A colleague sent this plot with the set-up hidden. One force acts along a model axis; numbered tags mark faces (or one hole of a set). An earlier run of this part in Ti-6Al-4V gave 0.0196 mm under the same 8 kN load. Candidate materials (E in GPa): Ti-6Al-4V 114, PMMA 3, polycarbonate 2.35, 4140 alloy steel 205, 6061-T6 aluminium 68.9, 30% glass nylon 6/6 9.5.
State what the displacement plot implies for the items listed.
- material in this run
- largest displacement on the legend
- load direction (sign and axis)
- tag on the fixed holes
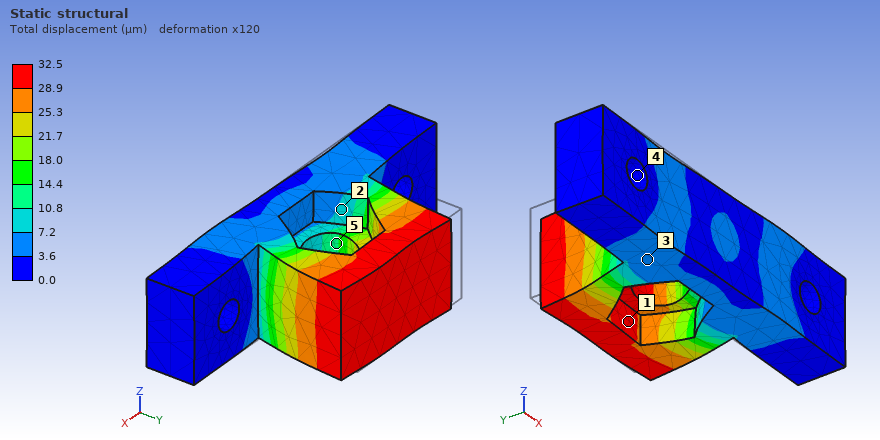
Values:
6061-T6 aluminium
32.5 µm
+X
4
